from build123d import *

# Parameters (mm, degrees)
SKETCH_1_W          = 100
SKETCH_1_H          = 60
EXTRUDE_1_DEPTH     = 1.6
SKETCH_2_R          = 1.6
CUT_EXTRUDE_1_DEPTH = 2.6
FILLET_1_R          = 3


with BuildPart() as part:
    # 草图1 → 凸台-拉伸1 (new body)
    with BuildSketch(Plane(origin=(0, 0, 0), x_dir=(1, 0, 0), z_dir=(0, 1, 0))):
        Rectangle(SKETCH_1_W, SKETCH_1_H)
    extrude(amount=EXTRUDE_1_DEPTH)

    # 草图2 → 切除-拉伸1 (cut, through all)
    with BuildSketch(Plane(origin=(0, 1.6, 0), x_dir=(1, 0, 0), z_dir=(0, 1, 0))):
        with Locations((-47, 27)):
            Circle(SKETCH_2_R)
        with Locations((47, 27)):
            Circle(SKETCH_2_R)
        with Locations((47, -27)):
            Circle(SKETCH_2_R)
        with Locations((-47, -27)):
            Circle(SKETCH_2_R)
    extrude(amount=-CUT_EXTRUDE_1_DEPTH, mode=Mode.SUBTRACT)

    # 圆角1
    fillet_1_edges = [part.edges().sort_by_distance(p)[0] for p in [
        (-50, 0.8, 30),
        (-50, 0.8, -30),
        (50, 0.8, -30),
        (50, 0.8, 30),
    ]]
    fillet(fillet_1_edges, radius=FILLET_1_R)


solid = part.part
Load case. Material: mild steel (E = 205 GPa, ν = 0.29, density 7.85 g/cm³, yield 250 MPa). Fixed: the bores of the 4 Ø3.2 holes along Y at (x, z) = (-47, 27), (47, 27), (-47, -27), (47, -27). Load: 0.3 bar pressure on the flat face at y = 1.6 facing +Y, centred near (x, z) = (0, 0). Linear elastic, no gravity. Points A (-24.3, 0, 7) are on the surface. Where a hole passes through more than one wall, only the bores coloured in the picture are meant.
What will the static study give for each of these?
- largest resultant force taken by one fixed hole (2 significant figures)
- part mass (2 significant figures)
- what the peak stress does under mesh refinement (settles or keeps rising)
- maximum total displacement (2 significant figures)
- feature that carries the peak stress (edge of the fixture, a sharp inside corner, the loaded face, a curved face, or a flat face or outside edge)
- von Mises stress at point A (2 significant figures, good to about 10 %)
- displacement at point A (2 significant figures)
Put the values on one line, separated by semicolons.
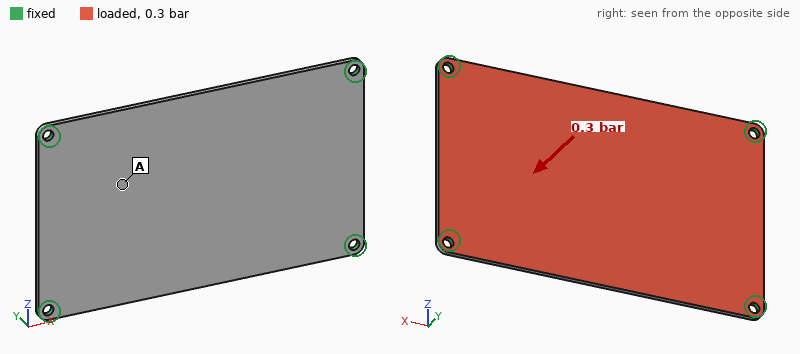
45 N; 75 g; keeps rising; 0.13 mm; edge of the fixture; 14 MPa; 0.086 mm
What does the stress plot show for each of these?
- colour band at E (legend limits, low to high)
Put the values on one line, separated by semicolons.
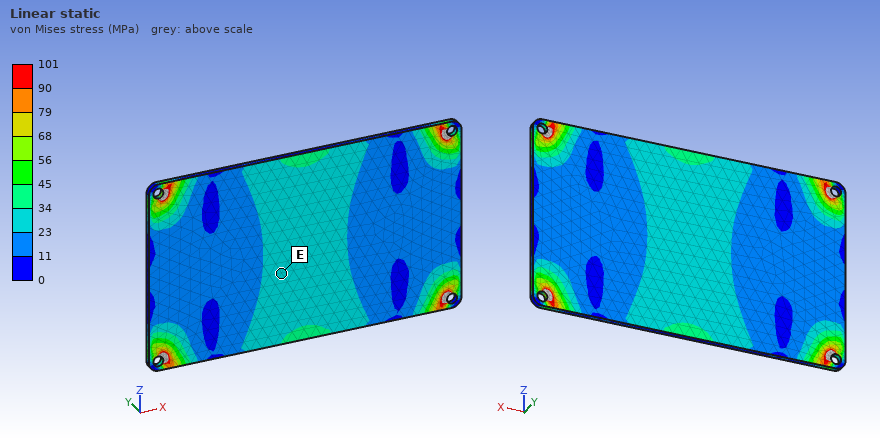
23 to 34 MPa
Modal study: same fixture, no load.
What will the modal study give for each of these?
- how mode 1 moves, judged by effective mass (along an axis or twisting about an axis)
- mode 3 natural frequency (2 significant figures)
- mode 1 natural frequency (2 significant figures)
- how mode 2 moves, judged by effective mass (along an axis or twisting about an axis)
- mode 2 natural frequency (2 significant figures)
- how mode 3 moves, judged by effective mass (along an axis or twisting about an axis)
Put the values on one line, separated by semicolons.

along Y; 2100 Hz; 770 Hz; twisting about X; 1400 Hz; twisting about Z
